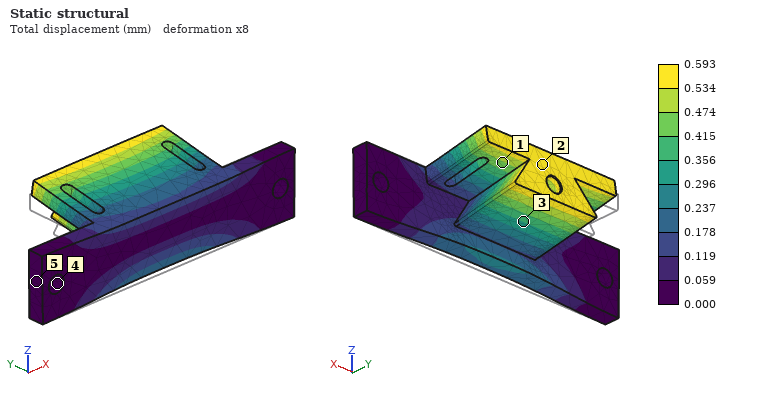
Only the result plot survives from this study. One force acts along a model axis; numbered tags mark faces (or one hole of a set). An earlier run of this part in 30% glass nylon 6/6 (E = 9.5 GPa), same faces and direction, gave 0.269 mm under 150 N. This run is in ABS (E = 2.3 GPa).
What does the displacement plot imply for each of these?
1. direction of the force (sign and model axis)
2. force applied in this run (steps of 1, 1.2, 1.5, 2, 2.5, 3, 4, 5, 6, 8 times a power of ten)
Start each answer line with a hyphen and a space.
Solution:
- +Z
- 80 N
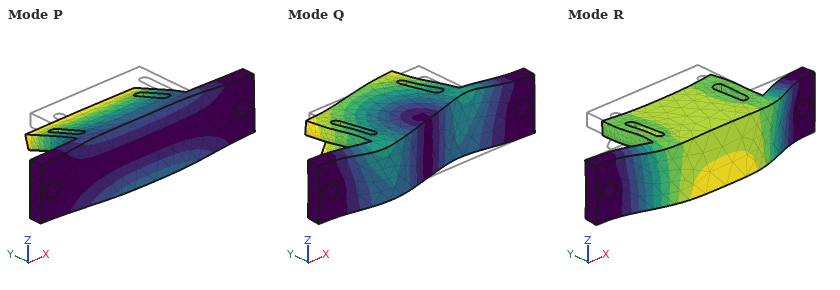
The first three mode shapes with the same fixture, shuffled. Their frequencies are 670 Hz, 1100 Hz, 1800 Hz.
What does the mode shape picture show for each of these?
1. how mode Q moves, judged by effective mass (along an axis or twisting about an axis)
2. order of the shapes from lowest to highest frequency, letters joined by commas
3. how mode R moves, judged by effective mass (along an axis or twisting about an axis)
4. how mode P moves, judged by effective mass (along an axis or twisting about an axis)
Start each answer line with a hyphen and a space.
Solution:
- along X
- P, R, Q
- along Y
- along Z
